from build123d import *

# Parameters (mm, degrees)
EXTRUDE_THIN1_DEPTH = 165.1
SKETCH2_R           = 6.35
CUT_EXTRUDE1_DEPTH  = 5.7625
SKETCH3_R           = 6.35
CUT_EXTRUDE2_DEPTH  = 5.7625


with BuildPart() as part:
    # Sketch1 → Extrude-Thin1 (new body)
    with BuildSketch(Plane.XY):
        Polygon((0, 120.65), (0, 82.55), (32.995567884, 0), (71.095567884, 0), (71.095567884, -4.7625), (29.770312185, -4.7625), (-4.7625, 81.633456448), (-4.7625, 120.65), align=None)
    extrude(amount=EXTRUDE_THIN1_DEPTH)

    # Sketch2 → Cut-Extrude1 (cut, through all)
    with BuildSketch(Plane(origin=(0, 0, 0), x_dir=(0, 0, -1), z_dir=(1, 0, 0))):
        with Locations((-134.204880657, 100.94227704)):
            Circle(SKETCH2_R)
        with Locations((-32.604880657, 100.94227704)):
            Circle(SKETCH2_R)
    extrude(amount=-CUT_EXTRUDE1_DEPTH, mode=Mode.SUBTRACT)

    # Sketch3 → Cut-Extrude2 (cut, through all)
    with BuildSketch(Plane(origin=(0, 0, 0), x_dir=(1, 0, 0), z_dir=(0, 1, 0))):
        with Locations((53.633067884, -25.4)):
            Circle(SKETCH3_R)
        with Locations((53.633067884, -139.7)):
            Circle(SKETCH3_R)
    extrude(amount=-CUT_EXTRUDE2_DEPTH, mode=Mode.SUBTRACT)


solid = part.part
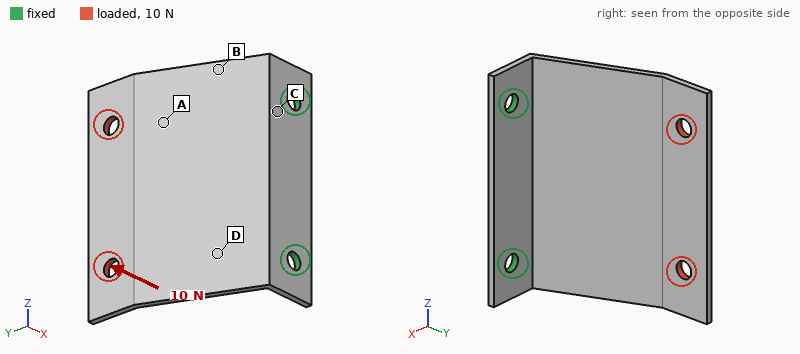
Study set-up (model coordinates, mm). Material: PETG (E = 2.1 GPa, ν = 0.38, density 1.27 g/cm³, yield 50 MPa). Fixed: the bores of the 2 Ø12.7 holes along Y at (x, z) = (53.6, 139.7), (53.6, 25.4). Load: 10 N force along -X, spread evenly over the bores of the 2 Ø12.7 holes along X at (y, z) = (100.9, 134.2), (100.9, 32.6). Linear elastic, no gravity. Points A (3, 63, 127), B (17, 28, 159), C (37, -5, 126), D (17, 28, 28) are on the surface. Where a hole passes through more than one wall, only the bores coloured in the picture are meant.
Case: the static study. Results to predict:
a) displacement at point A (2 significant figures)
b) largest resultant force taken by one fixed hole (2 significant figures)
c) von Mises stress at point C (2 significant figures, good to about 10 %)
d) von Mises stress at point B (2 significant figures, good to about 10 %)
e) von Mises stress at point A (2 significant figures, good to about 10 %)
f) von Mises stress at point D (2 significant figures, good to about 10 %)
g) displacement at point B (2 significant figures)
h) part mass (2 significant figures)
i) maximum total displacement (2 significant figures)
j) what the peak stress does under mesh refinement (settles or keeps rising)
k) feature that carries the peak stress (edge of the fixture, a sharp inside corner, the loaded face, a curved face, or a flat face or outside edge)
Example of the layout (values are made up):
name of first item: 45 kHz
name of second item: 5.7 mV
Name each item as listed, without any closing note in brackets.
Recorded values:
displacement at point A: 1.1 mm
largest resultant force taken by one fixed hole: 6.1 N
von Mises stress at point C: 1.6 MPa
von Mises stress at point B: 1.2 MPa
von Mises stress at point A: 0.52 MPa
von Mises stress at point D: 1.0 MPa
displacement at point B: 0.41 mm
part mass: 170 g
maximum total displacement: 2.5 mm
what the peak stress does under mesh refinement: keeps rising
feature that carries the peak stress: edge of the fixture
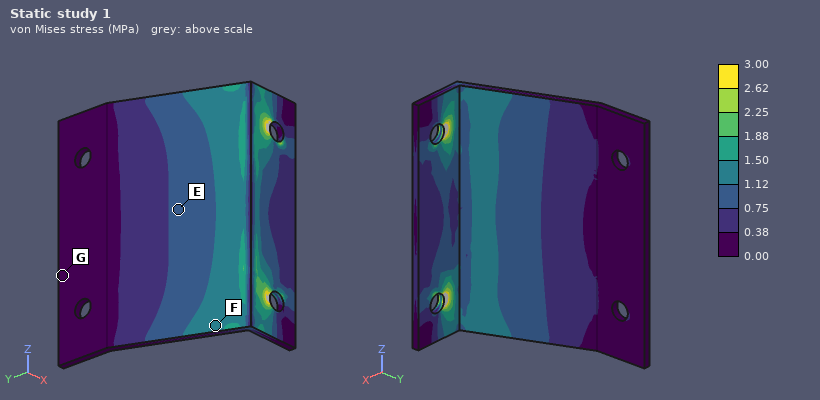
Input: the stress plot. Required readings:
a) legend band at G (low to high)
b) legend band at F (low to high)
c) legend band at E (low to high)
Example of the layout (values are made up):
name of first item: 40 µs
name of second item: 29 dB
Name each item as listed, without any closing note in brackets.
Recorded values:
legend band at G: 0.00 to 0.38 MPa
legend band at F: 1.12 to 1.50 MPa
legend band at E: 0.75 to 1.12 MPa
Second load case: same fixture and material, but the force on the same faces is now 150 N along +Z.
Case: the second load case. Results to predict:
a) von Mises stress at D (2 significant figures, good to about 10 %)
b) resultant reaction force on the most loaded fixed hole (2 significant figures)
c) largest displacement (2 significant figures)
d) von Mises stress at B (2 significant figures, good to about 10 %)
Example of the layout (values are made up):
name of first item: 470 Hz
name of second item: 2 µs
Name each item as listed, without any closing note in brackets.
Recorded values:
von Mises stress at D: 1.4 MPa
resultant reaction force on the most loaded fixed hole: 170 N
largest displacement: 2.5 mm
von Mises stress at B: 1.7 MPa
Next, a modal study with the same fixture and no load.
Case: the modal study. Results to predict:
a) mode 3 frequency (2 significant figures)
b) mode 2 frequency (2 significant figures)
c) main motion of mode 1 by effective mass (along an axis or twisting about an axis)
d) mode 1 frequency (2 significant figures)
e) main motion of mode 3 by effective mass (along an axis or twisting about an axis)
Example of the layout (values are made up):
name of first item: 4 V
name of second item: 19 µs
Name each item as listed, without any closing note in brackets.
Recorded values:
mode 3 frequency: 280 Hz
mode 2 frequency: 110 Hz
main motion of mode 1 by effective mass: along X
mode 1 frequency: 47 Hz
main motion of mode 3 by effective mass: along Y
